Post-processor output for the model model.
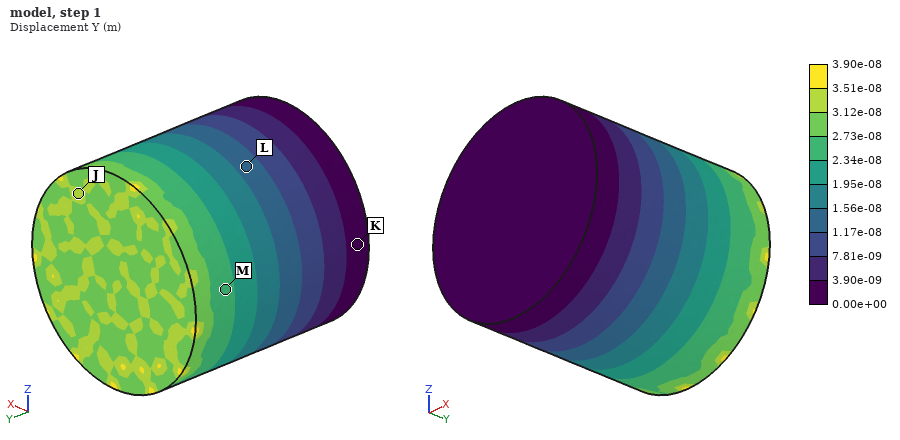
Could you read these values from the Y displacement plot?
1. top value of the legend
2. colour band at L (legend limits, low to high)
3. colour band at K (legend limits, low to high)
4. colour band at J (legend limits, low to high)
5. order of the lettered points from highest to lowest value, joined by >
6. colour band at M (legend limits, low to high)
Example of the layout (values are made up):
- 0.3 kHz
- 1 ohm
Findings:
- 3.90e-08 m
- 1.17e-08 to 1.56e-08 m
- 0.00e+00 to 3.90e-09 m
- 3.12e-08 to 3.51e-08 m
- J > M > L > K
- 2.34e-08 to 2.73e-08 m
